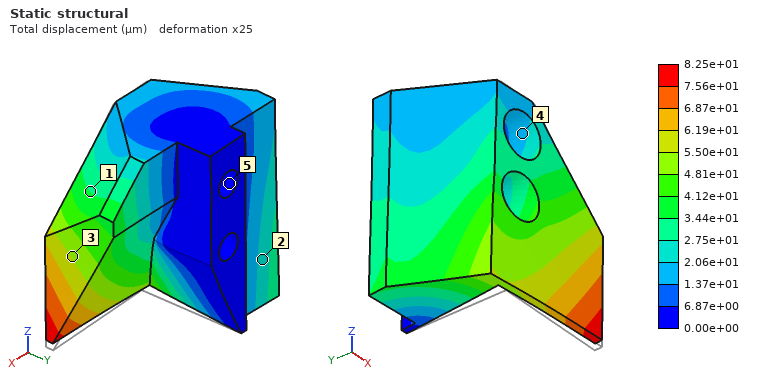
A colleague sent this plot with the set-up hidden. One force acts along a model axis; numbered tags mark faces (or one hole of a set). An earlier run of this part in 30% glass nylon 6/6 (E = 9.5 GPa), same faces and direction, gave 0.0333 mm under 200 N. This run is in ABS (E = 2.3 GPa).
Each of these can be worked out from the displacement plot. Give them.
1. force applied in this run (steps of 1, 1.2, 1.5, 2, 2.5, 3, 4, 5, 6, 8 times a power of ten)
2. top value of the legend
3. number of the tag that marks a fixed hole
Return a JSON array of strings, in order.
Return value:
["120 N", "8.25e+01 µm", "5"]
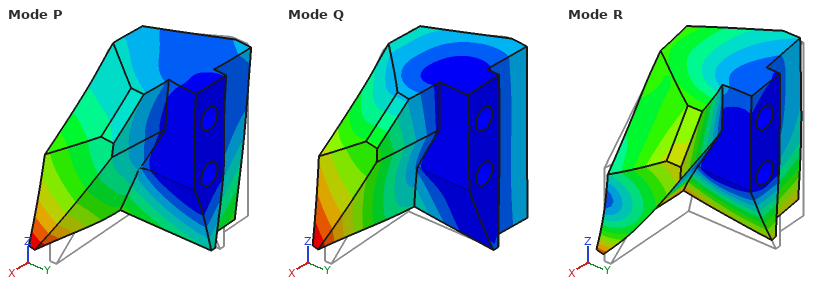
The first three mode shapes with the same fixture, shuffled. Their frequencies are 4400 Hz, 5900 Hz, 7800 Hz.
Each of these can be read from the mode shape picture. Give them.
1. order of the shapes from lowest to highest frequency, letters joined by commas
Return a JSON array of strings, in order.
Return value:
["Q, P, R"]
